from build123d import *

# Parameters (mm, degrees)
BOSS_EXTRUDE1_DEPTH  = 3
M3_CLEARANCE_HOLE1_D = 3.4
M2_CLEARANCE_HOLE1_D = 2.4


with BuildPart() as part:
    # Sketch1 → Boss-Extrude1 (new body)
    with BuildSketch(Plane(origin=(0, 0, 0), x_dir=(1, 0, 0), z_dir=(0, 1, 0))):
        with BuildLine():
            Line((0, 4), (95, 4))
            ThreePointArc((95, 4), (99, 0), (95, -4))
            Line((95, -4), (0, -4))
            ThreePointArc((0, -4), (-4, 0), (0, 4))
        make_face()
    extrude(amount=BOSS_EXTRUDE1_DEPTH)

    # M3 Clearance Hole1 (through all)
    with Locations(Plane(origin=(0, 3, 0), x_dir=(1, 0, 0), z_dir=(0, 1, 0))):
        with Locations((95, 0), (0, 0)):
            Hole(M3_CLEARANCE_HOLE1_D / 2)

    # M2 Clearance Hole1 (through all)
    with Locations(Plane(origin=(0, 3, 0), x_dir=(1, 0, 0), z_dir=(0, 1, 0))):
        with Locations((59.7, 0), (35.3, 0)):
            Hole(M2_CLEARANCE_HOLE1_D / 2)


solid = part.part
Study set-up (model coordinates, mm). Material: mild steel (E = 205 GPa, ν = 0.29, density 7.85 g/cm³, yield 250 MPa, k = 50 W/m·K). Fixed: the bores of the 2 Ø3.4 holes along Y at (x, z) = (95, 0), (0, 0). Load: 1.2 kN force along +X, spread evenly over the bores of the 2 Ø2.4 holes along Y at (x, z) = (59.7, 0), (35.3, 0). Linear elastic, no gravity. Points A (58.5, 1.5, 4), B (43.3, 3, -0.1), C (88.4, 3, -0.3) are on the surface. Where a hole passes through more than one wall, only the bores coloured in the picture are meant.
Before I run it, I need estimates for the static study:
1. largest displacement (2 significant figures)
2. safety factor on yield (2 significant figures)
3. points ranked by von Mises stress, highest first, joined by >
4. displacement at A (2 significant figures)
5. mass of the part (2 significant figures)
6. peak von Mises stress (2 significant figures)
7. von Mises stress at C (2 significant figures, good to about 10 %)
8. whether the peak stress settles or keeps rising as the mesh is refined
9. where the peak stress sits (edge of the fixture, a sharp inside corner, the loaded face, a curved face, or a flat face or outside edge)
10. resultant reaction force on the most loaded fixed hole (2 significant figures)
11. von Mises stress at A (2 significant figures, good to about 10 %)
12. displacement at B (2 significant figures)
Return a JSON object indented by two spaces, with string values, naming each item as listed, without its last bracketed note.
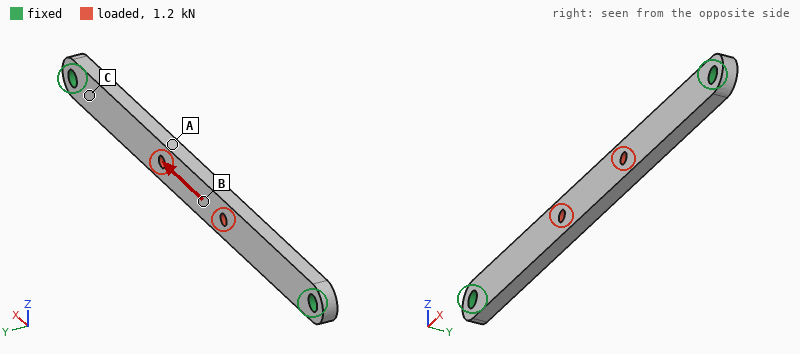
{
  "largest displacement": "4.7 µm",
  "safety factor on yield": "4.0",
  "points ranked by von Mises stress, highest first, joined by >": "C > A > B",
  "displacement at A": "4.2 µm",
  "mass of the part": "18 g",
  "peak von Mises stress": "62 MPa",
  "von Mises stress at C": "27 MPa",
  "whether the peak stress settles or keeps rising as the mesh is refined": "settles",
  "where the peak stress sits": "the loaded face",
  "resultant reaction force on the most loaded fixed hole": "600 N",
  "von Mises stress at A": "13 MPa",
  "displacement at B": "4.4 µm"
}
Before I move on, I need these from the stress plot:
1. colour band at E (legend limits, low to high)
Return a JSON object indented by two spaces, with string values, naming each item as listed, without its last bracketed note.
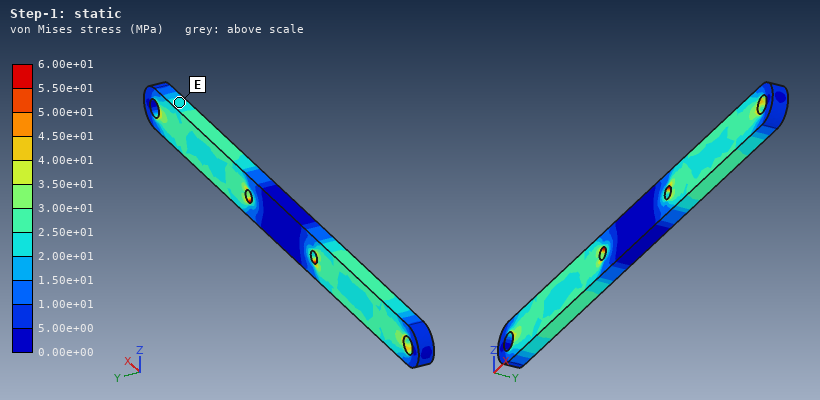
{
  "colour band at E": "2.00e+01 to 2.50e+01 MPa"
}
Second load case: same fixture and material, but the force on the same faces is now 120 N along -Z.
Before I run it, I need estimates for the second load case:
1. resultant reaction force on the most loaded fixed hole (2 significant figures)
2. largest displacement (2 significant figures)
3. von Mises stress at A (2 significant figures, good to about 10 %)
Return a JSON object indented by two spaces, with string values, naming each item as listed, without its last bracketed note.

{
  "resultant reaction force on the most loaded fixed hole": "60 N",
  "largest displacement": "20 µm",
  "von Mises stress at A": "28 MPa"
}
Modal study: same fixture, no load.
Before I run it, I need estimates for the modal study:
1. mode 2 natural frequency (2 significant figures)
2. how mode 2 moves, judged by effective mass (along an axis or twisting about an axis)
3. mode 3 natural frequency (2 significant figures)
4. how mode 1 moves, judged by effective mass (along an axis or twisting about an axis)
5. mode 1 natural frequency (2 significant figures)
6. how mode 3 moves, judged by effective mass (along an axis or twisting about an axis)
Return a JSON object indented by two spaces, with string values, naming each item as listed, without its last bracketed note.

{
  "mode 2 natural frequency": "4300 Hz",
  "how mode 2 moves, judged by effective mass": "along Z",
  "mode 3 natural frequency": "4900 Hz",
  "how mode 1 moves, judged by effective mass": "along Y",
  "mode 1 natural frequency": "1800 Hz",
  "how mode 3 moves, judged by effective mass": "twisting about Z"
}
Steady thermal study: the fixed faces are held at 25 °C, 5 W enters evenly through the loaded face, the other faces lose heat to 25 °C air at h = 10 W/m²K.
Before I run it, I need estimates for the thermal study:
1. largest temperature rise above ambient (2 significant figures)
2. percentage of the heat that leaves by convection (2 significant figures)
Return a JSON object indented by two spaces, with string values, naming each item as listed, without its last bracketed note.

{
  "largest temperature rise above ambient": "65 K",
  "percentage of the heat that leaves by convection": "16 %"
}
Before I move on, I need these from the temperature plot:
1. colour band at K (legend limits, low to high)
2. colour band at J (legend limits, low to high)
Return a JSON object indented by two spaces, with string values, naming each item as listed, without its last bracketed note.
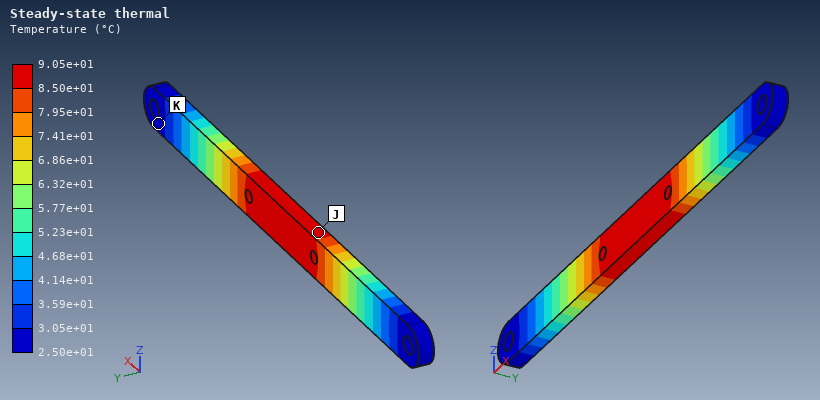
{
  "colour band at K": "2.50e+01 to 3.05e+01 °C",
  "colour band at J": "8.50e+01 to 9.05e+01 °C"
}
